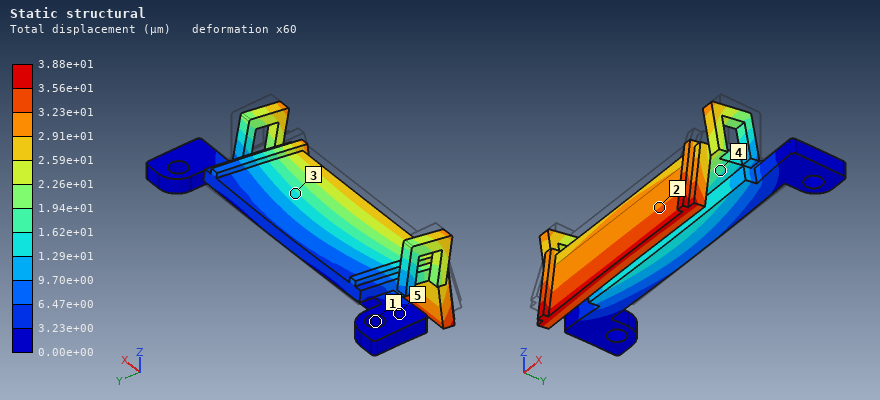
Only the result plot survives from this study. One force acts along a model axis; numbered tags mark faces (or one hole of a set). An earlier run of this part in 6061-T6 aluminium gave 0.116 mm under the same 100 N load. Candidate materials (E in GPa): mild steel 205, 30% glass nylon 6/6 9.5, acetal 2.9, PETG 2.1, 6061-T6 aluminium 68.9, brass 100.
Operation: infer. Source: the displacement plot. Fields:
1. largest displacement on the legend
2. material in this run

3.88e+01 µm
mild steel
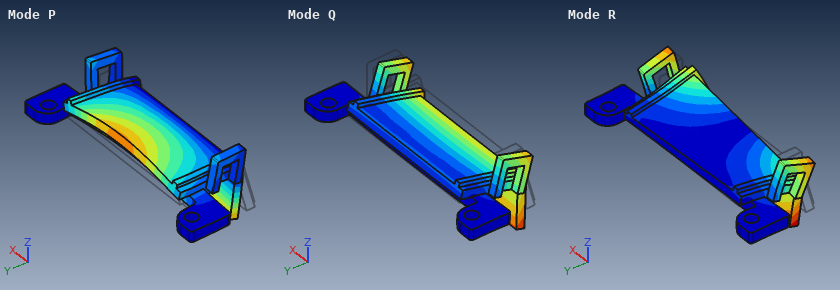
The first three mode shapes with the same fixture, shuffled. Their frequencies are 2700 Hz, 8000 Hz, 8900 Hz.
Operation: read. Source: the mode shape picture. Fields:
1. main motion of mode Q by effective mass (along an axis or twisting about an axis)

along Z
